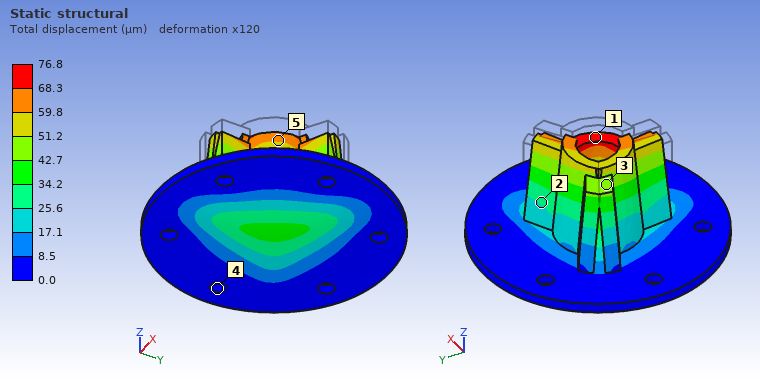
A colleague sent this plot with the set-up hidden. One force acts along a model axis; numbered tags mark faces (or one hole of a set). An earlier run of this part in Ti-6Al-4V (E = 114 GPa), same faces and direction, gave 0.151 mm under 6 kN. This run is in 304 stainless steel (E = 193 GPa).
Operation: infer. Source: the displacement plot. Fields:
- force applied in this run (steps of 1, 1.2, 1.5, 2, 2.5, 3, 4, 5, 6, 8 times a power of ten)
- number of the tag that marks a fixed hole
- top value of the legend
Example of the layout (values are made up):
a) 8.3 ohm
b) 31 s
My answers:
a) 5 kN
b) 4
c) 76.8 µm
